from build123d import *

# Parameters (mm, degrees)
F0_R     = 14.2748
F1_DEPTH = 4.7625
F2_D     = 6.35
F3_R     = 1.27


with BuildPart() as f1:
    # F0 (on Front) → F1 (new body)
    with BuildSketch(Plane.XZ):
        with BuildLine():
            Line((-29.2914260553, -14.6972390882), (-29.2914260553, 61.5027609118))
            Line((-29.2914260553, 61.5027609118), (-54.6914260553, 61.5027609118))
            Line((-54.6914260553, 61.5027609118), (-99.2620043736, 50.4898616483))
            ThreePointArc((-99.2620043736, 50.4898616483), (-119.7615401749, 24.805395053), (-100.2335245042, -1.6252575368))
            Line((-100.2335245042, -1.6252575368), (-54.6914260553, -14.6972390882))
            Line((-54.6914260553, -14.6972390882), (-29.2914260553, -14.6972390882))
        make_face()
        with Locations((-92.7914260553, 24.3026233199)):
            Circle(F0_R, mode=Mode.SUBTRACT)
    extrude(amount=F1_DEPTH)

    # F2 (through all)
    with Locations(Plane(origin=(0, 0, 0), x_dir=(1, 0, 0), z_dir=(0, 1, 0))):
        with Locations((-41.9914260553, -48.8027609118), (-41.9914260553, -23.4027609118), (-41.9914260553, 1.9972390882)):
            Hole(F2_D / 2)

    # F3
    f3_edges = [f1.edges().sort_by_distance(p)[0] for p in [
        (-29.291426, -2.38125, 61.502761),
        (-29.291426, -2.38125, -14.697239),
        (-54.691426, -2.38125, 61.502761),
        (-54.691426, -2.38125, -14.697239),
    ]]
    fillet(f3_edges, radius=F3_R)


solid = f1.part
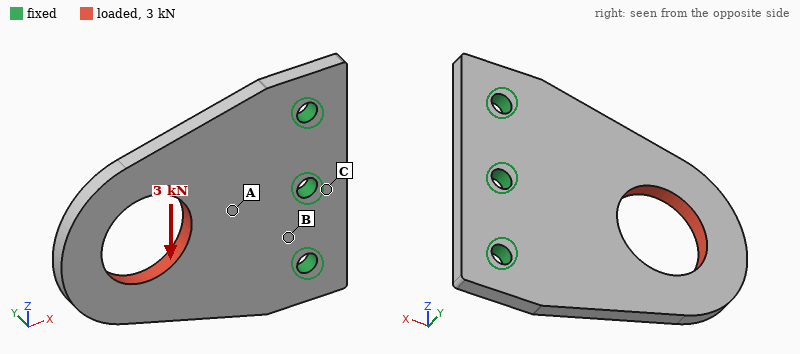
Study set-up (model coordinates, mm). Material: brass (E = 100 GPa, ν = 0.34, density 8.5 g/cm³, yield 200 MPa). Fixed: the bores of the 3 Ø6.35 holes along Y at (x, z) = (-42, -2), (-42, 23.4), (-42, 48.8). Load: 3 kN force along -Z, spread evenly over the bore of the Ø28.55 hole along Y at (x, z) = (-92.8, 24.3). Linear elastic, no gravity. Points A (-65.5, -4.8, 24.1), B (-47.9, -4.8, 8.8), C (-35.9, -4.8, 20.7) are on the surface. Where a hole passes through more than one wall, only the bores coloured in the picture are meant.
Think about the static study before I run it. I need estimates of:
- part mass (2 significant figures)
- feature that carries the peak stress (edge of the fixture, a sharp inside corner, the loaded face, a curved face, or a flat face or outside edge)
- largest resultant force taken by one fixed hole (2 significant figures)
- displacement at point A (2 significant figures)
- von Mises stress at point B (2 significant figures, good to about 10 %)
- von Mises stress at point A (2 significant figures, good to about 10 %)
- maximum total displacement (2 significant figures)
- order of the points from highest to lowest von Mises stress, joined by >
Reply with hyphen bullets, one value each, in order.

- 200 g
- edge of the fixture
- 2.9 kN
- 9.4 µm
- 18 MPa
- 31 MPa
- 49 µm
- A > B > C
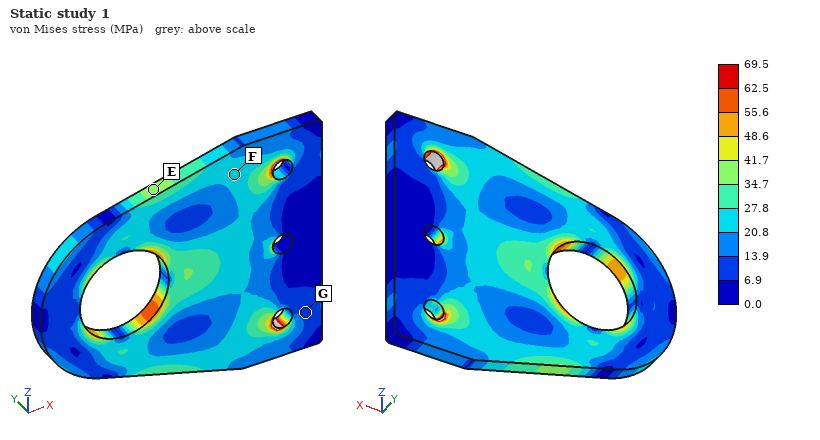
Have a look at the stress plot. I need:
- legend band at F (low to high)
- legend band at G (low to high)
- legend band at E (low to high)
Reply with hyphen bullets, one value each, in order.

- 20.8 to 27.8 MPa
- 6.9 to 13.9 MPa
- 34.7 to 41.7 MPa
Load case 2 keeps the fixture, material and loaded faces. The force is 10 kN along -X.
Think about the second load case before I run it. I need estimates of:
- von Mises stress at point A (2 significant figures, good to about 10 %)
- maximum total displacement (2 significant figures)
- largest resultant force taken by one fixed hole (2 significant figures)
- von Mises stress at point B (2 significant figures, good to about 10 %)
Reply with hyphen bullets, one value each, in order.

- 27 MPa
- 39 µm
- 3.7 kN
- 17 MPa
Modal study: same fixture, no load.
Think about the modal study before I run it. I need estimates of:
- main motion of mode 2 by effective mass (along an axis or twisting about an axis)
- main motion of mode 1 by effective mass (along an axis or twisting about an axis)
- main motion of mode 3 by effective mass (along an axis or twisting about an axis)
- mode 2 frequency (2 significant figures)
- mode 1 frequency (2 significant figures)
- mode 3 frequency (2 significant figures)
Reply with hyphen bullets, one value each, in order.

- twisting about X
- along Y
- along Y
- 1700 Hz
- 650 Hz
- 2700 Hz
